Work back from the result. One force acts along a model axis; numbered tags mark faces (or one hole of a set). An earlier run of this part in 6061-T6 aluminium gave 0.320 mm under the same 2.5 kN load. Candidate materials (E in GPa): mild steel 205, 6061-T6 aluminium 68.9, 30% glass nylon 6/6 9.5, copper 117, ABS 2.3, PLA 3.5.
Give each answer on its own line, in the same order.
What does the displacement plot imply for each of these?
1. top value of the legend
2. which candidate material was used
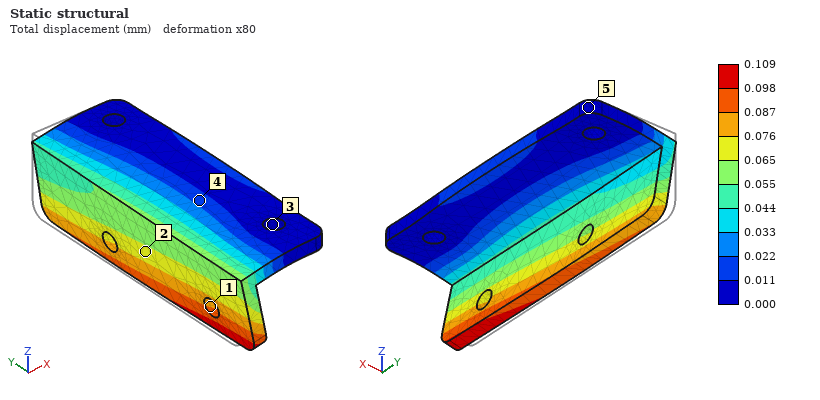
0.109 mm
mild steel
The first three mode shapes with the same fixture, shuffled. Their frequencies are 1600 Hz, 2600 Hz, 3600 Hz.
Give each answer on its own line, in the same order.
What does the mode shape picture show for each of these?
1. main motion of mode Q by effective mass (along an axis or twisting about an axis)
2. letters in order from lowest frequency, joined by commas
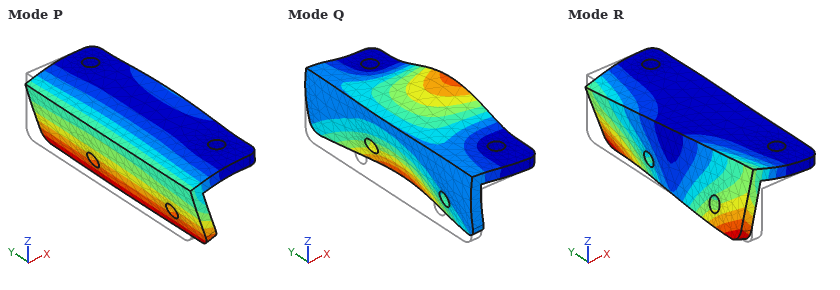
along Z
P, R, Q
